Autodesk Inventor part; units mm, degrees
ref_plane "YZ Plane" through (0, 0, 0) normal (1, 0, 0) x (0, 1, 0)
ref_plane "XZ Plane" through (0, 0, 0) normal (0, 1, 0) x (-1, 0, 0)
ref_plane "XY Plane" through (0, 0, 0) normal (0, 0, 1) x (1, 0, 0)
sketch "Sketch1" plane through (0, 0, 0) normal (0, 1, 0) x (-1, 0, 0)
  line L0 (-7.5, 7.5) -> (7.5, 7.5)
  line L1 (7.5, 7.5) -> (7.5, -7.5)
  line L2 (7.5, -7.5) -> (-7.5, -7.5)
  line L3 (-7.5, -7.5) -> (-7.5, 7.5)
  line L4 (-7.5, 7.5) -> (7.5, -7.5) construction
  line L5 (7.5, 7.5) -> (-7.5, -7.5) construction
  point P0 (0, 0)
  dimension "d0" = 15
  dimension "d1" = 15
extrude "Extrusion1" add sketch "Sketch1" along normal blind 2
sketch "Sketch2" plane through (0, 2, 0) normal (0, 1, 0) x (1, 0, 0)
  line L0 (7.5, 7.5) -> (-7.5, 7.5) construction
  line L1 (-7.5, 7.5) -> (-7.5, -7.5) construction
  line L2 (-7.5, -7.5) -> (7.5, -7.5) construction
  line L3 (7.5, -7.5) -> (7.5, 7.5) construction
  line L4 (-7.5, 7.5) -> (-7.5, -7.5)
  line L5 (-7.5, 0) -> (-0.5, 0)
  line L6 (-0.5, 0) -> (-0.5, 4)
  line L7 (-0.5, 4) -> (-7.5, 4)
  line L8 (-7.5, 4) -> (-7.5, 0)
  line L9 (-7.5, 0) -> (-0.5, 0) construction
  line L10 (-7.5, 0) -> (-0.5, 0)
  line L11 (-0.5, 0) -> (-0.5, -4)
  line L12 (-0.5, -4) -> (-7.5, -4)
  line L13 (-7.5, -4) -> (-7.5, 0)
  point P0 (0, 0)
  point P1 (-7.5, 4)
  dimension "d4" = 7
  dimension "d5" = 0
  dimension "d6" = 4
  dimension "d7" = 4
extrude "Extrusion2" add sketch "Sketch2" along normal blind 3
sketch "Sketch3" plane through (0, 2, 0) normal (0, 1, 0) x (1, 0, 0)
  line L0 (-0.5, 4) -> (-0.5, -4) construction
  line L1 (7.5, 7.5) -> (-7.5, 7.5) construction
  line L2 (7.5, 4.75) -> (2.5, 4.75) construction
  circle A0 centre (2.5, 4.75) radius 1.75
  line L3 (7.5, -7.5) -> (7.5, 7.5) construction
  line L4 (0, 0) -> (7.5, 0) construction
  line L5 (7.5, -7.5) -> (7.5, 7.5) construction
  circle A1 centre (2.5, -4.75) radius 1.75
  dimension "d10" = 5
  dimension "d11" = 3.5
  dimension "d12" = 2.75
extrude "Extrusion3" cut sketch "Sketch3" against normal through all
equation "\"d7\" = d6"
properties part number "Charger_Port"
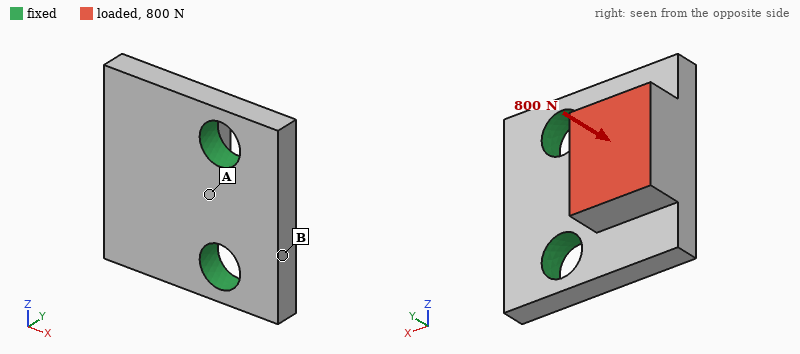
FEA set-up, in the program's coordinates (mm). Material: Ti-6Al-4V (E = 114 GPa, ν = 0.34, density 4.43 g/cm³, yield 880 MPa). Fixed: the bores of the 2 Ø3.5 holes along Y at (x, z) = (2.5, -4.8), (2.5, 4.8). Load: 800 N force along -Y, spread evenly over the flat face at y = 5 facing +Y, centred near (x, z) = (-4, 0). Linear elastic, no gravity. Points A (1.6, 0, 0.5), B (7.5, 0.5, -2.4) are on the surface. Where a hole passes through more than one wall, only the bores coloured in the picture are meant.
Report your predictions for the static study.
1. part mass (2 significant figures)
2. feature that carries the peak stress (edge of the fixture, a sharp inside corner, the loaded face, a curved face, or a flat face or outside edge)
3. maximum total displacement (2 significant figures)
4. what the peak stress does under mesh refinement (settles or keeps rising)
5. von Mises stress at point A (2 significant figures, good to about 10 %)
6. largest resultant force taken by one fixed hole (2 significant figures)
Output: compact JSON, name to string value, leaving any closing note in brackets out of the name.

{"part mass": "2.6 g", "feature that carries the peak stress": "edge of the fixture", "maximum total displacement": "78 µm", "what the peak stress does under mesh refinement": "keeps rising", "von Mises stress at point A": "160 MPa", "largest resultant force taken by one fixed hole": "400 N"}
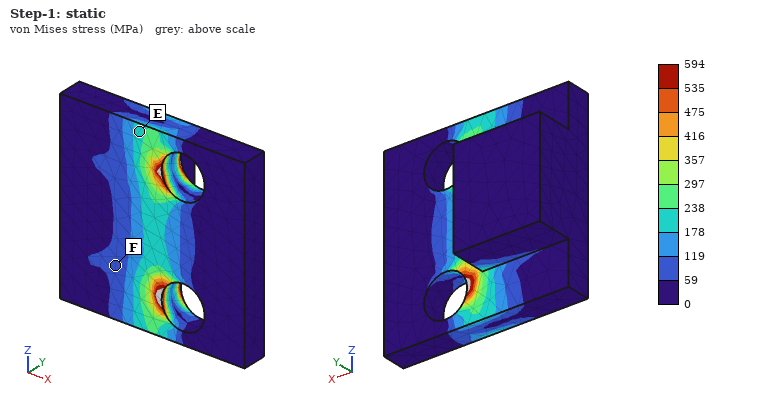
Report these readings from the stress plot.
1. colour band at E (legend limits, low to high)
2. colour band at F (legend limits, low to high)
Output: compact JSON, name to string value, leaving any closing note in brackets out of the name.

{"colour band at E": "178 to 238 MPa", "colour band at F": "59 to 119 MPa"}
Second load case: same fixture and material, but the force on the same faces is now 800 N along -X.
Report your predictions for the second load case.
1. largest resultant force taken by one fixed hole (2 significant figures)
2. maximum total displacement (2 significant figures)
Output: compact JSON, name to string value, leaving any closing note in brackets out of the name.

{"largest resultant force taken by one fixed hole": "420 N", "maximum total displacement": "75 µm"}
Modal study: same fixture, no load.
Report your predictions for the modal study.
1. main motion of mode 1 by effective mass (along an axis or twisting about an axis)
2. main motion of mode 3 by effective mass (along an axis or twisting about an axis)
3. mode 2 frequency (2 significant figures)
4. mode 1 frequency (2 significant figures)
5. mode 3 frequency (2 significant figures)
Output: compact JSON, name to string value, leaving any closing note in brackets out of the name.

{"main motion of mode 1 by effective mass": "along Y", "main motion of mode 3 by effective mass": "along Z", "mode 2 frequency": "42 kHz", "mode 1 frequency": "15 kHz", "mode 3 frequency": "56 kHz"}
